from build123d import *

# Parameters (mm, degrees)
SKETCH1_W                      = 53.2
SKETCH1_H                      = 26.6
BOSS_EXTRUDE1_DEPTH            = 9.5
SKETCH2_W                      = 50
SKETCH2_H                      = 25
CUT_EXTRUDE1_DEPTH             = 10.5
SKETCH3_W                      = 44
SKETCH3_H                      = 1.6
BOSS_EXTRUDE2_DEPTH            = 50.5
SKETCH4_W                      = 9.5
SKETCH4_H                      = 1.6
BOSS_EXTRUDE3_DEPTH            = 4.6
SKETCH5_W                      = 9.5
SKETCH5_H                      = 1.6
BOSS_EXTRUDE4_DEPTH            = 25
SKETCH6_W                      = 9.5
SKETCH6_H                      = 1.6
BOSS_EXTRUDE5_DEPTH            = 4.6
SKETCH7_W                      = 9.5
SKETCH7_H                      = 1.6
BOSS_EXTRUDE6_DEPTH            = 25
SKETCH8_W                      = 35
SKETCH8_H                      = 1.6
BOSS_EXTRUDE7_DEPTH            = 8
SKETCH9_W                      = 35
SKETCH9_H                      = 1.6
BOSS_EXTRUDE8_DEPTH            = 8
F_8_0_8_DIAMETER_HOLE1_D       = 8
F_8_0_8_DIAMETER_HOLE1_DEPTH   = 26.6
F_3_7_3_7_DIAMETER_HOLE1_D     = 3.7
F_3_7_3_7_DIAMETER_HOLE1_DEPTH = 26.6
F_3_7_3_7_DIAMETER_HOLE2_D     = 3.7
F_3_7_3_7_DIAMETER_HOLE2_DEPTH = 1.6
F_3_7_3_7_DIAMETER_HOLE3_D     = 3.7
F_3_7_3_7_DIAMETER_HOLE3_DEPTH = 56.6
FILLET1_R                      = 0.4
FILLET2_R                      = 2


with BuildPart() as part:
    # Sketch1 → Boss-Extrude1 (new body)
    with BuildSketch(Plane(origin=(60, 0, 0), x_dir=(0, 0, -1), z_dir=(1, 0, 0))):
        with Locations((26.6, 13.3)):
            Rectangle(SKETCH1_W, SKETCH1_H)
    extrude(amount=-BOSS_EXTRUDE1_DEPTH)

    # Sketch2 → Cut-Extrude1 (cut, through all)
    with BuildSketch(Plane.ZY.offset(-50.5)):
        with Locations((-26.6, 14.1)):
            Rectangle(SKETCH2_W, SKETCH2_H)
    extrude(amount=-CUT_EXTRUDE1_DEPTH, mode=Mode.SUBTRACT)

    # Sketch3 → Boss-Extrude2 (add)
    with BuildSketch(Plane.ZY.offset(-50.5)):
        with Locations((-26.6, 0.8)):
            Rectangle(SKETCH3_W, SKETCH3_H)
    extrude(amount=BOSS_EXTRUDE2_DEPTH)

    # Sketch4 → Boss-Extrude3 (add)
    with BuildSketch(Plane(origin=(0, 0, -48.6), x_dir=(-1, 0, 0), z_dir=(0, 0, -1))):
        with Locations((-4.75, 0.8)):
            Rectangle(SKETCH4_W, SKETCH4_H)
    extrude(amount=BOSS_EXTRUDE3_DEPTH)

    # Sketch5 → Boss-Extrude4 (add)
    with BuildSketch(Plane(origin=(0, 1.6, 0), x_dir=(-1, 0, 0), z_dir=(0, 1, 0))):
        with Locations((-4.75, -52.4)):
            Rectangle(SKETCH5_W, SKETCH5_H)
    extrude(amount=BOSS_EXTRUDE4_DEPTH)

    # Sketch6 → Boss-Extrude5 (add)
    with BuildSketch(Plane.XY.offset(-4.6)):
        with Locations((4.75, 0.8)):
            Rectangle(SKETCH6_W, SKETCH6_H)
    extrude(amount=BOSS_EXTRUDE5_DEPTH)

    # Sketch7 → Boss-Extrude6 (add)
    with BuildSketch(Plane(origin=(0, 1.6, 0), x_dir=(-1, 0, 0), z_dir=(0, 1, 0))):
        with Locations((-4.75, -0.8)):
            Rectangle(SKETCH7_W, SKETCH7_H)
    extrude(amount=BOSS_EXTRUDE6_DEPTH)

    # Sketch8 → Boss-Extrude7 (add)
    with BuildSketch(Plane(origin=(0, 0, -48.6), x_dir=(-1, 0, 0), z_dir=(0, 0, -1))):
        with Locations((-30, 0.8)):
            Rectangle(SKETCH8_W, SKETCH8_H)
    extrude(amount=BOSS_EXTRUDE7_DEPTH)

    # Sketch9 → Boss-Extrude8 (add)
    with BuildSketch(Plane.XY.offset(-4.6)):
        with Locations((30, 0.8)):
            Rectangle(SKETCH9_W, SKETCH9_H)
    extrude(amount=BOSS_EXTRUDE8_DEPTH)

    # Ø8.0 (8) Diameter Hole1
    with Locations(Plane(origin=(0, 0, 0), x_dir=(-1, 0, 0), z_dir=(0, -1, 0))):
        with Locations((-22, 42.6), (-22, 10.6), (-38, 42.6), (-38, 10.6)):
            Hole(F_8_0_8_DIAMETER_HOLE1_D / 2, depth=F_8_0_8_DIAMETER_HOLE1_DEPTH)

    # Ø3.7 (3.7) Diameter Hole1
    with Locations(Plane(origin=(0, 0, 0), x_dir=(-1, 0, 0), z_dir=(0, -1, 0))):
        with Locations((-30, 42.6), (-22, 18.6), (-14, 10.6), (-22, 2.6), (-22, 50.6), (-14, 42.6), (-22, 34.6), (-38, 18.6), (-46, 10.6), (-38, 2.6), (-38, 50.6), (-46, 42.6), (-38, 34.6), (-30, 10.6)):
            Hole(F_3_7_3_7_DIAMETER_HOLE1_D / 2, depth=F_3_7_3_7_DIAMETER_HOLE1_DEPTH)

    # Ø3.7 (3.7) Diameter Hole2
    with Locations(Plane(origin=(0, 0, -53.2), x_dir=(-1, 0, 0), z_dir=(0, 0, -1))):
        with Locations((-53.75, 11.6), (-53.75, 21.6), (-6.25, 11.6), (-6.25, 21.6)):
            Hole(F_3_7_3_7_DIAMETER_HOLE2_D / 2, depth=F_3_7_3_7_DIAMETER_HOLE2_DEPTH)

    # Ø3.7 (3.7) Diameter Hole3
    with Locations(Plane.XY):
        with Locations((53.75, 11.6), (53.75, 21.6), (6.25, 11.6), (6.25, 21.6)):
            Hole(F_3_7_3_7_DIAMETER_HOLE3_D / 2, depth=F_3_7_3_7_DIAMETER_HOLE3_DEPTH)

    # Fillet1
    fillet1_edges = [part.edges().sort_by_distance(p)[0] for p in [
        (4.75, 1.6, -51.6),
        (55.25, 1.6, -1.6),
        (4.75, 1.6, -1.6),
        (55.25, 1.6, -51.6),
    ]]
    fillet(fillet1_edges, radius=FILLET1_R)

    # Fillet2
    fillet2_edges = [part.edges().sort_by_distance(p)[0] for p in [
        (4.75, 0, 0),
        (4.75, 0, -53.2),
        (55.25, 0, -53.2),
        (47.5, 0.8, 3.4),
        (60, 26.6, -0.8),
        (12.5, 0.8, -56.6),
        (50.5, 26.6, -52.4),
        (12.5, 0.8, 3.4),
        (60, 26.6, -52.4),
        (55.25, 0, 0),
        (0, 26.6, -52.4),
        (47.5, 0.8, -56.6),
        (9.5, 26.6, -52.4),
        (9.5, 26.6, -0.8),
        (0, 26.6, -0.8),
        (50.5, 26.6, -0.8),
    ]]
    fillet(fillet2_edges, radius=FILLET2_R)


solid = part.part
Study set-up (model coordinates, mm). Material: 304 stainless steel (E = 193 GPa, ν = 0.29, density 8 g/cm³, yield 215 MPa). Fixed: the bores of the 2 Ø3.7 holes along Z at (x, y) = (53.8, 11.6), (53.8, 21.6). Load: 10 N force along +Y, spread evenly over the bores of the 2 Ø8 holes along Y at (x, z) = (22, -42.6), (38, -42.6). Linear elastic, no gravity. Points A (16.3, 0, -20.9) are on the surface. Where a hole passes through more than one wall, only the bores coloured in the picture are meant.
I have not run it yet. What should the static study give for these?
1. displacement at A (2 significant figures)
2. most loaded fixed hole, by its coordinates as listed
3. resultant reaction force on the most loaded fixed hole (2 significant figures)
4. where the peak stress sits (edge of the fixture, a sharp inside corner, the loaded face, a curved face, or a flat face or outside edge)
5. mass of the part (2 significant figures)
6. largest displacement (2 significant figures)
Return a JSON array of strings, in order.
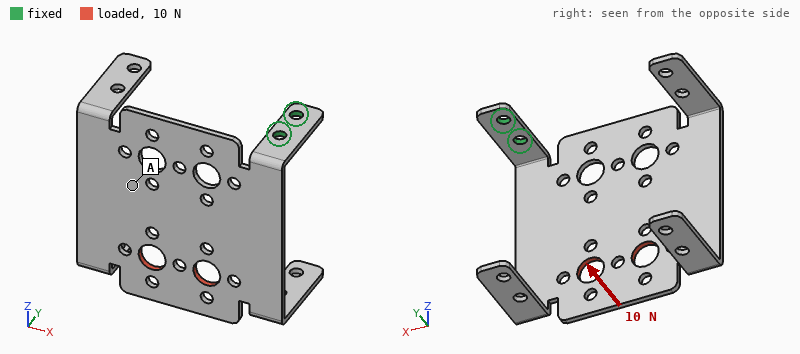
["0.38 mm", "(53.8, 11.6)", "22 N", "a curved face", "49 g", "0.98 mm"]
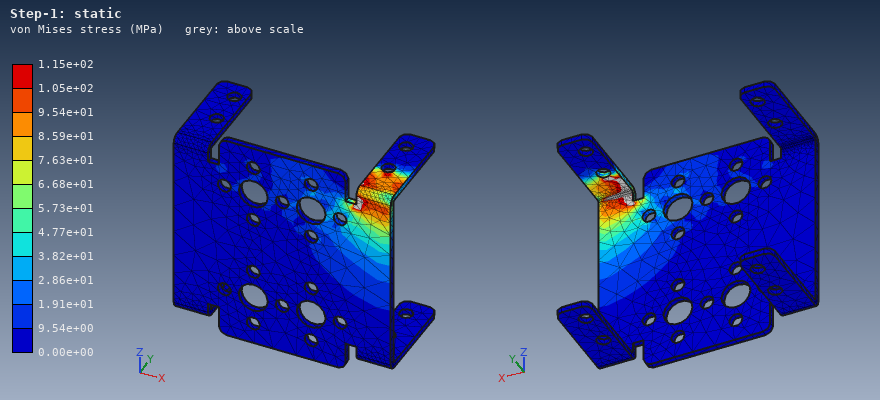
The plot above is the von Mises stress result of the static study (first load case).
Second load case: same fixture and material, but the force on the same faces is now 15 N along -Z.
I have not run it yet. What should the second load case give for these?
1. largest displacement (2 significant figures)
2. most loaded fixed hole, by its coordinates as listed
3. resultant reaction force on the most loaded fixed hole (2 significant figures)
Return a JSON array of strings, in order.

["0.28 mm", "(53.8, 11.6)", "12 N"]
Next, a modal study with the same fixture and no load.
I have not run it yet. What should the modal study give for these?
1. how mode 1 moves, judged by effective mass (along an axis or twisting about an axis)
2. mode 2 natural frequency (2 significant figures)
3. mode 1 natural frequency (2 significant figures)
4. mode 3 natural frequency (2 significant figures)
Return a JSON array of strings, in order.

["along Y", "160 Hz", "110 Hz", "240 Hz"]
